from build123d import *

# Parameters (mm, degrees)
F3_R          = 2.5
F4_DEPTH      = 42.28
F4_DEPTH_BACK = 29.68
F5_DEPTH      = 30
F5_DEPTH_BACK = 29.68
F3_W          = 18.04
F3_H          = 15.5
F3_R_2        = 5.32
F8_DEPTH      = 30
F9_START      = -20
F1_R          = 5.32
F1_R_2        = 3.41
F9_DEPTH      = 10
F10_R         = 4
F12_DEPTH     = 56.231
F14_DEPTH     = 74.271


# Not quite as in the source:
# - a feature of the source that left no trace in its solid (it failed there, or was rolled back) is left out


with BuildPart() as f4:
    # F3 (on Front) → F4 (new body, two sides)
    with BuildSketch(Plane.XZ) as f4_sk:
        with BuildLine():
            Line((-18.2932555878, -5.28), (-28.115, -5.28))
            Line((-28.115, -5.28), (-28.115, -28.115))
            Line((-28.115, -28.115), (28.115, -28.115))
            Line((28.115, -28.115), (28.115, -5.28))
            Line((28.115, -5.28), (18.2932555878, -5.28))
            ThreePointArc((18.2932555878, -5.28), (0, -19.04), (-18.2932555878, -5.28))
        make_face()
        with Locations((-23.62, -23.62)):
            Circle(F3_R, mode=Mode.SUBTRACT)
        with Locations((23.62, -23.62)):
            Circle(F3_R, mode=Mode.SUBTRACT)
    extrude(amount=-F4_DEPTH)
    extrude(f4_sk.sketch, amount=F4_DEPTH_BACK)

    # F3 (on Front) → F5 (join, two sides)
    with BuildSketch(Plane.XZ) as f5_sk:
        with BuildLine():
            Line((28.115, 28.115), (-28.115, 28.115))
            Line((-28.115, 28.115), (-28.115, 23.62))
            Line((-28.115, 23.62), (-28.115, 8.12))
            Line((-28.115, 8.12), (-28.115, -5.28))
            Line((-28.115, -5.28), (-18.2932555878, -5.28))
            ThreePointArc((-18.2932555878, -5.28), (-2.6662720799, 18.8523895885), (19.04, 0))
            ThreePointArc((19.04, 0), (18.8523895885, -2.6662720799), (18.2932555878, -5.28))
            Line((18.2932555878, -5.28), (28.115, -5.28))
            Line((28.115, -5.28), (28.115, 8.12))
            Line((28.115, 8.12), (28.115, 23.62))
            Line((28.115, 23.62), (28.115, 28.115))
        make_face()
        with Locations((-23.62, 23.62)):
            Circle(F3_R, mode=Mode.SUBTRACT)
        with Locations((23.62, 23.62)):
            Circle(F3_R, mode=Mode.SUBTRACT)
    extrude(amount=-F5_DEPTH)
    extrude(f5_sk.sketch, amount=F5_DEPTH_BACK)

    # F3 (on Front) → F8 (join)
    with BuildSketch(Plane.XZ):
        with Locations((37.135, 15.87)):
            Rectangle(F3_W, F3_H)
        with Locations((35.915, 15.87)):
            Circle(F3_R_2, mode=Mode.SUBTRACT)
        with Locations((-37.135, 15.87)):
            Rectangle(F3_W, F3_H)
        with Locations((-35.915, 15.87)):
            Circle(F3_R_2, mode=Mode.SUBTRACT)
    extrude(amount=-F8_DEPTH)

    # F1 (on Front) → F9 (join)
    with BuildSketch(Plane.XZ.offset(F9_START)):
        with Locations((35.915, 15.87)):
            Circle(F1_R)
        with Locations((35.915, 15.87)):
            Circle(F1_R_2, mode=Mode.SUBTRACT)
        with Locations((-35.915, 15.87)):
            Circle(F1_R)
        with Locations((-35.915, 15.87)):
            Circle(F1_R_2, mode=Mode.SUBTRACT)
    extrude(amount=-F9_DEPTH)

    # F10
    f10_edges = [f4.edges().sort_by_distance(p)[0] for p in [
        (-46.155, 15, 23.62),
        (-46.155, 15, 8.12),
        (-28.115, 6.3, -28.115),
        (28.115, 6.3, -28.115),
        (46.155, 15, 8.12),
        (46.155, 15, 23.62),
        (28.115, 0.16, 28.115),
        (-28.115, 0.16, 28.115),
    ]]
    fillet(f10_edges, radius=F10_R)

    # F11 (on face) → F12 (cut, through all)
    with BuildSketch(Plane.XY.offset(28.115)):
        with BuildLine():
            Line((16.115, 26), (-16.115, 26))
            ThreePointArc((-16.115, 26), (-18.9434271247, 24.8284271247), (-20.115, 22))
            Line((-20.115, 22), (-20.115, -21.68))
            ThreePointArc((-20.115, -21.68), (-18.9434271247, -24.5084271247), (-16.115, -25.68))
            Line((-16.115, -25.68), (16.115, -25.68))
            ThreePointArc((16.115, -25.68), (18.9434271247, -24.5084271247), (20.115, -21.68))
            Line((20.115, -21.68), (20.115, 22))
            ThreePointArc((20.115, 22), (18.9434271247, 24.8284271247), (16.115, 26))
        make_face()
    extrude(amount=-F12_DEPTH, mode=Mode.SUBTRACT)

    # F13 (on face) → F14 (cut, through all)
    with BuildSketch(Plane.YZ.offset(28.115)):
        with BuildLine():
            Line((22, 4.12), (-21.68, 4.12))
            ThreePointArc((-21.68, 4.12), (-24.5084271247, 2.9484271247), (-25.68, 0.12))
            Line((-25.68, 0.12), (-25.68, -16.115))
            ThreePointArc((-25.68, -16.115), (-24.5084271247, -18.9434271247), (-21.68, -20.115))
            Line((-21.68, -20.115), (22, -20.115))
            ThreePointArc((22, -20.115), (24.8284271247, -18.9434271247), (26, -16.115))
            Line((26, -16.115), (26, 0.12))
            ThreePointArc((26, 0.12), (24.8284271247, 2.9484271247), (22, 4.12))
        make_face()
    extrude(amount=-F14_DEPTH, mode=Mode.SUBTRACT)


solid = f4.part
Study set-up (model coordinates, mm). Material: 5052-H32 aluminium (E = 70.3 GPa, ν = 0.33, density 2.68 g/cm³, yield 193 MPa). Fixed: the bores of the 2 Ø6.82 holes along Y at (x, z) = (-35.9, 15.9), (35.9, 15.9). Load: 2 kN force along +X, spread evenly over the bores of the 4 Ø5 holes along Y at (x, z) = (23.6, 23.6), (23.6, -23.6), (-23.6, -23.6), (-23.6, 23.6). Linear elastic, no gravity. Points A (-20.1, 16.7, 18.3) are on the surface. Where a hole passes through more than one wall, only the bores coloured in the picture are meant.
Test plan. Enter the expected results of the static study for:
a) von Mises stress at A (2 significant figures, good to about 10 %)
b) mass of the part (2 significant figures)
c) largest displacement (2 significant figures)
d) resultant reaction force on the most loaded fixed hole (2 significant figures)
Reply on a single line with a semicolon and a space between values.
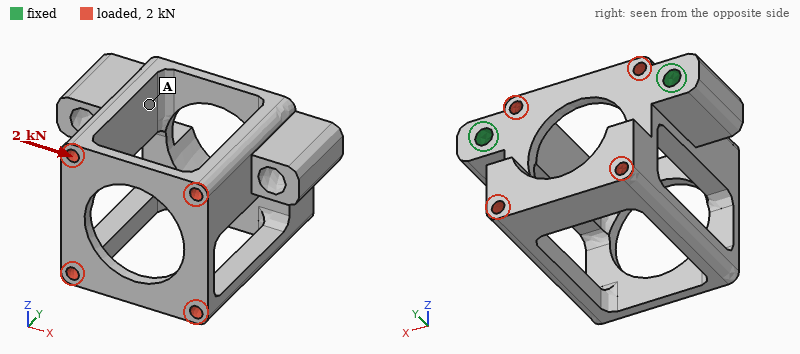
6.6 MPa; 160 g; 100 µm; 1.2 kN
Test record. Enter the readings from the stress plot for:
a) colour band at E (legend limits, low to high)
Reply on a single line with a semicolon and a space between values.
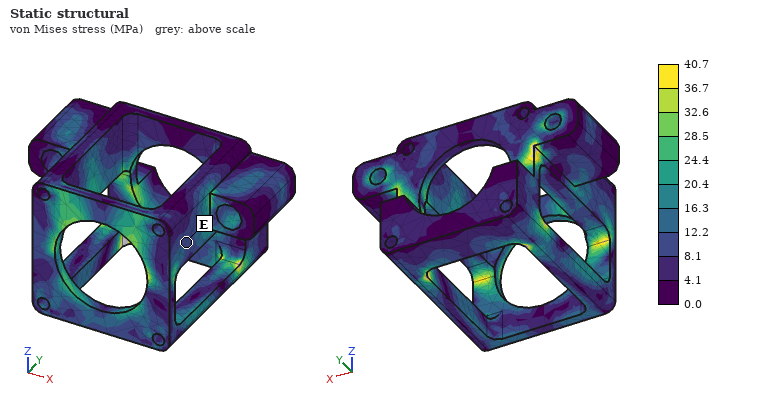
8.1 to 12.2 MPa
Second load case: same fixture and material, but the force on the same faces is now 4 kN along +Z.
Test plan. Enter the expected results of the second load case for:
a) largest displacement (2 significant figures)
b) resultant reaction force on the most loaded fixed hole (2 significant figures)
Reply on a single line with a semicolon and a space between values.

0.18 mm; 2.0 kN
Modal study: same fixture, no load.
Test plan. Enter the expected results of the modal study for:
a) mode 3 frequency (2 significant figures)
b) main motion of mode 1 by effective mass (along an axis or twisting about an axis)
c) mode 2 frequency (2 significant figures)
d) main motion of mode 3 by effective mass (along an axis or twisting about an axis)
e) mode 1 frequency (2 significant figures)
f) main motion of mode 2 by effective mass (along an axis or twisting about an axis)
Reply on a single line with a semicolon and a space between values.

3600 Hz; along Y; 2700 Hz; along Z; 1700 Hz; along X
